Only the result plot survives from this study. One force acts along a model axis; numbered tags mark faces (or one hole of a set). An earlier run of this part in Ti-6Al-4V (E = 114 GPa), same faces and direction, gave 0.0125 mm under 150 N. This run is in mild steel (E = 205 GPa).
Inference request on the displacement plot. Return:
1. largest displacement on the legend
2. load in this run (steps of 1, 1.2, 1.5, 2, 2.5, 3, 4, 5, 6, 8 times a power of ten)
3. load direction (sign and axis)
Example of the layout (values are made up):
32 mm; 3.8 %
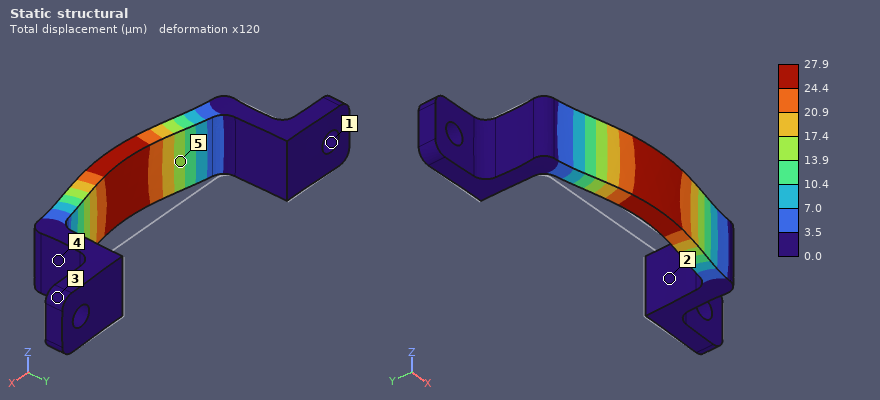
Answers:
27.9 µm; 600 N; -Y
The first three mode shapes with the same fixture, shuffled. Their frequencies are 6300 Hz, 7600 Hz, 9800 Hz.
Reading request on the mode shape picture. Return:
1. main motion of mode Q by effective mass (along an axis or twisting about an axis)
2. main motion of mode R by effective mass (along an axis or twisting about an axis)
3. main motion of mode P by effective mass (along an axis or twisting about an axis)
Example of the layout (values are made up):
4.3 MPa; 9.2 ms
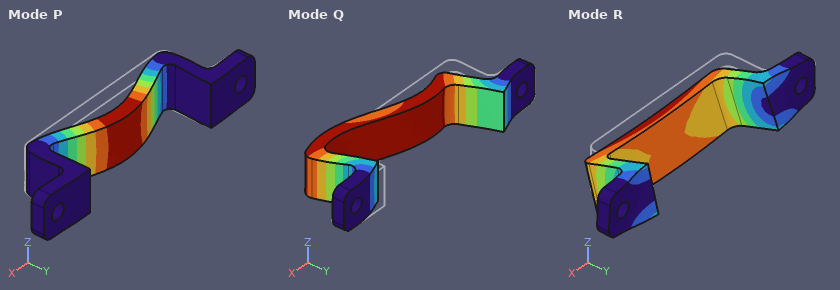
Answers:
along X; along Z; along Y
